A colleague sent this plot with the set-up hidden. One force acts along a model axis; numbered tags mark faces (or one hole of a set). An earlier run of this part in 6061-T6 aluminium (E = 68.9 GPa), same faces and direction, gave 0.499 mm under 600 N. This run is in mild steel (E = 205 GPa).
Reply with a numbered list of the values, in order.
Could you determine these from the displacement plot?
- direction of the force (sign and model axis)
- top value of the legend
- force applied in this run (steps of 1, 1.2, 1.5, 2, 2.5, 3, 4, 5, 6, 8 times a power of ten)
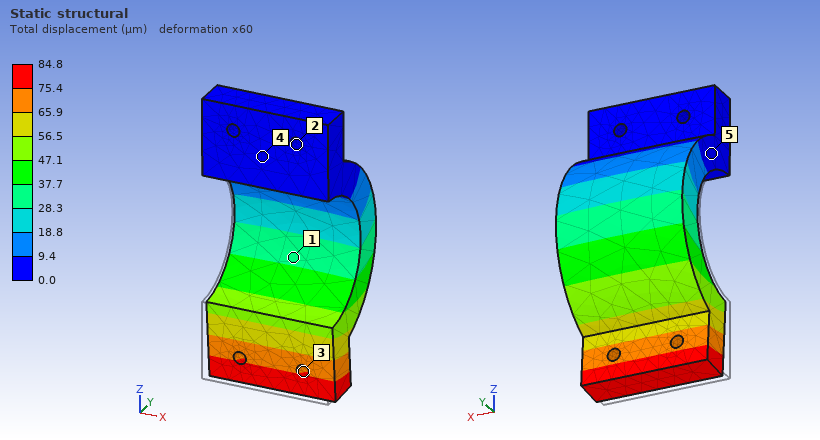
1. +Y
2. 84.8 µm
3. 300 N
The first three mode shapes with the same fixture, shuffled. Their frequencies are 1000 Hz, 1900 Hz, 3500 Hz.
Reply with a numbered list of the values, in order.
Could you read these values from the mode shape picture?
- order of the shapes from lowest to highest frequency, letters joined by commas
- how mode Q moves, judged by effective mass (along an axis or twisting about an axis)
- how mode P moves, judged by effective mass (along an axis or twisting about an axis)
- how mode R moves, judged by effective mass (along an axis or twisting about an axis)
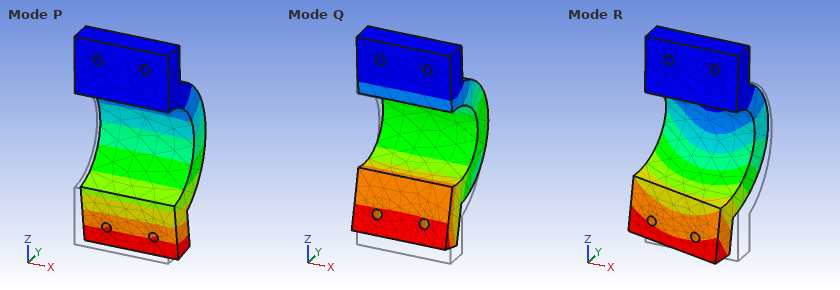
1. P, R, Q
2. along Z
3. along Y
4. along X
